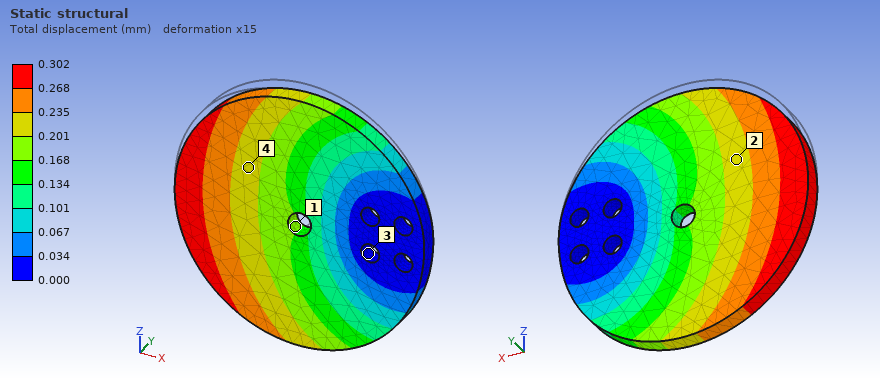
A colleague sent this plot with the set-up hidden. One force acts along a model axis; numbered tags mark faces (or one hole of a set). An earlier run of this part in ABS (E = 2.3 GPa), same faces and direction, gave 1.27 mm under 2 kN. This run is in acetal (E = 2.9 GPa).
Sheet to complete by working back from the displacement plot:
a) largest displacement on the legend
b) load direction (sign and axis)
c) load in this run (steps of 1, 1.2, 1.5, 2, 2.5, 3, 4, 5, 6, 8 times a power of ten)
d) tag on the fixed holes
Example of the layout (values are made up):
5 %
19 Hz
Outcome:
0.302 mm
-Z
600 N
3
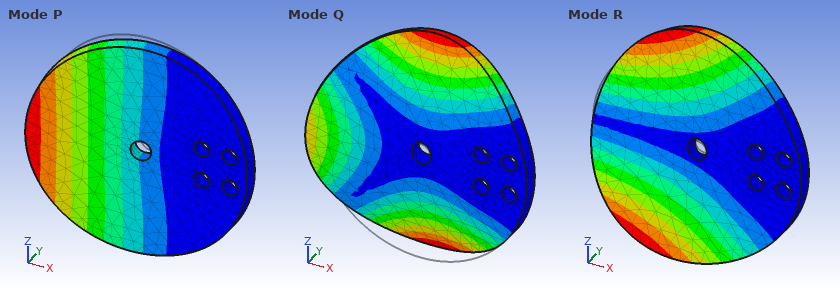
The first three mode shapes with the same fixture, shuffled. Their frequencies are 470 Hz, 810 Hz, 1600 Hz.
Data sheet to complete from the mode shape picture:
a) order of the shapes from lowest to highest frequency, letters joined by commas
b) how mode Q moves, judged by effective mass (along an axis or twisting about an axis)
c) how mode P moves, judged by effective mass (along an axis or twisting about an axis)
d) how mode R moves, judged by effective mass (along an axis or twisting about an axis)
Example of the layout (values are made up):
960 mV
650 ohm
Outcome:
P, R, Q
along Y
along Y
twisting about X
